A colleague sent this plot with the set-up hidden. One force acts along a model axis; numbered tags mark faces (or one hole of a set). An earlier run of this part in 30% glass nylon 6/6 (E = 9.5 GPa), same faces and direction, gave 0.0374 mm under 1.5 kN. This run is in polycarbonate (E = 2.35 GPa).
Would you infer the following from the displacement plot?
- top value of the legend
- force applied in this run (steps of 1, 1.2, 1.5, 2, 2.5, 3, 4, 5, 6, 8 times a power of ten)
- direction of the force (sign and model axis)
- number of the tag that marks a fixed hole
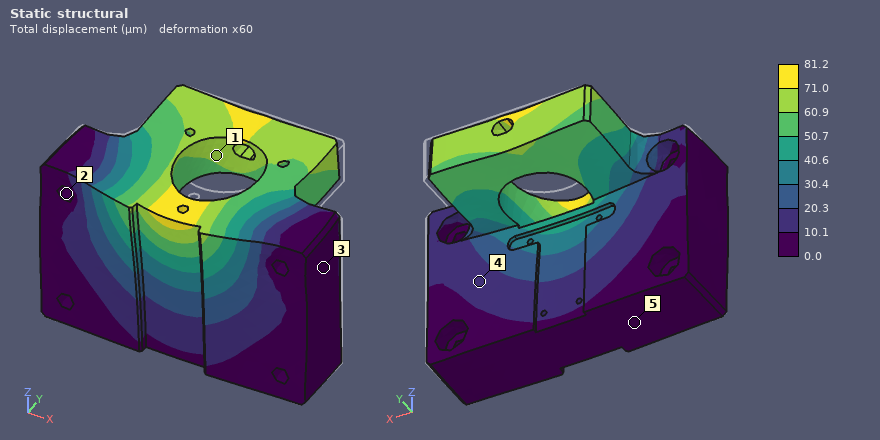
81.2 µm
800 N
-Y
2
